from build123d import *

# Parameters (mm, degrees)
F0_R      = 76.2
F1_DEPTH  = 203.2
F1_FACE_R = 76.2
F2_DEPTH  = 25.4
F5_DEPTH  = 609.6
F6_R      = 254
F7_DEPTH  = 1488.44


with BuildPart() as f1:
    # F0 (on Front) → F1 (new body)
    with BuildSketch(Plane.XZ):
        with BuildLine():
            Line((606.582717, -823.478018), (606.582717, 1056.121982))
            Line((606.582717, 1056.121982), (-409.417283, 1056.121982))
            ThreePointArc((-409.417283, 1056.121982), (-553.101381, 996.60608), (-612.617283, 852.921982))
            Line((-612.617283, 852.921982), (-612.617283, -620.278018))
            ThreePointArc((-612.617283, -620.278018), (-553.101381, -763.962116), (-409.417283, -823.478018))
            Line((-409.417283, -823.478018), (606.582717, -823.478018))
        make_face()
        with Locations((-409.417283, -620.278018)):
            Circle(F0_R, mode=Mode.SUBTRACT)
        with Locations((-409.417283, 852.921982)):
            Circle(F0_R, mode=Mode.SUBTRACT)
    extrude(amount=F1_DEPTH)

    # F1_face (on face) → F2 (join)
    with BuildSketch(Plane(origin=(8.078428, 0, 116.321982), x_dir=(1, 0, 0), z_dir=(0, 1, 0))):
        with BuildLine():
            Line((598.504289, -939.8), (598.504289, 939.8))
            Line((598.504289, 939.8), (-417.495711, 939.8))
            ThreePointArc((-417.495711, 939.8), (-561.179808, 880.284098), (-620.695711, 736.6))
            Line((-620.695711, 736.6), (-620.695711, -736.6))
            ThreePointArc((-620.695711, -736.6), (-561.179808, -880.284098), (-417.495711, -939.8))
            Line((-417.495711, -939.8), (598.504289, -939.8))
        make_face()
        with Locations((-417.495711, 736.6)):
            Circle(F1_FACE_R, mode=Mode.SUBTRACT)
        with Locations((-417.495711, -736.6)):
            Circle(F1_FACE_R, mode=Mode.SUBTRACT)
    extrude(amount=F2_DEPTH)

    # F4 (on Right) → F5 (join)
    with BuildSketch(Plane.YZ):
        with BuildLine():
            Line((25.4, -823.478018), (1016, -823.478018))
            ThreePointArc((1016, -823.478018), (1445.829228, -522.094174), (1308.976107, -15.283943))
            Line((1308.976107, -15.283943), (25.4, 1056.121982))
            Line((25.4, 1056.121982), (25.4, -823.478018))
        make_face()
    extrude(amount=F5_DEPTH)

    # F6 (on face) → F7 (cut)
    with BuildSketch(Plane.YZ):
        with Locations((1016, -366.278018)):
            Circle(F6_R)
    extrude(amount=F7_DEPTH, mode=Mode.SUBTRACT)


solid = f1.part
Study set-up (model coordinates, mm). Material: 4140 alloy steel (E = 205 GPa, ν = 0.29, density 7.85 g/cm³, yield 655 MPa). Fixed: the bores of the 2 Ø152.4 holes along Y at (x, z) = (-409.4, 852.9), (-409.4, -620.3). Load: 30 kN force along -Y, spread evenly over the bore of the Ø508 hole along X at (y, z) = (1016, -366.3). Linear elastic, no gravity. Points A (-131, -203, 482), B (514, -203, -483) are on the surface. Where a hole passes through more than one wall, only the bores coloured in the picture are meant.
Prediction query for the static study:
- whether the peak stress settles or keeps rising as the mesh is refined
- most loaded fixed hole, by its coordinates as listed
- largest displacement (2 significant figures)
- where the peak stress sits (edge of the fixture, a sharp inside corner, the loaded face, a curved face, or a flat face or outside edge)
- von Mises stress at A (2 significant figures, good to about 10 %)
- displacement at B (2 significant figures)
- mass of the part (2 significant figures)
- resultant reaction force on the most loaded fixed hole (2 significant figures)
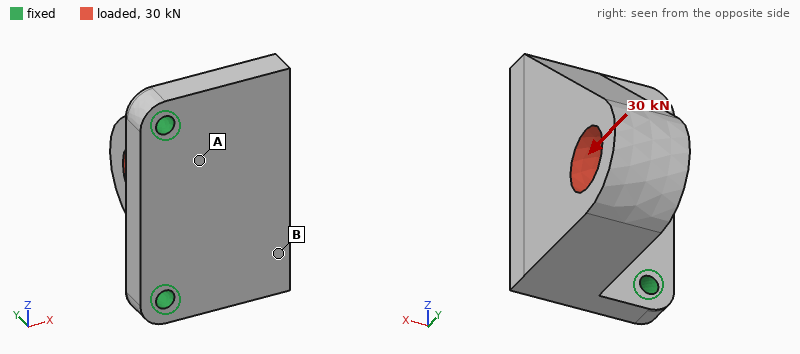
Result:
keeps rising
(-409.4, -620.3)
46 µm
edge of the fixture
0.60 MPa
21 µm
12000 kg
25 kN
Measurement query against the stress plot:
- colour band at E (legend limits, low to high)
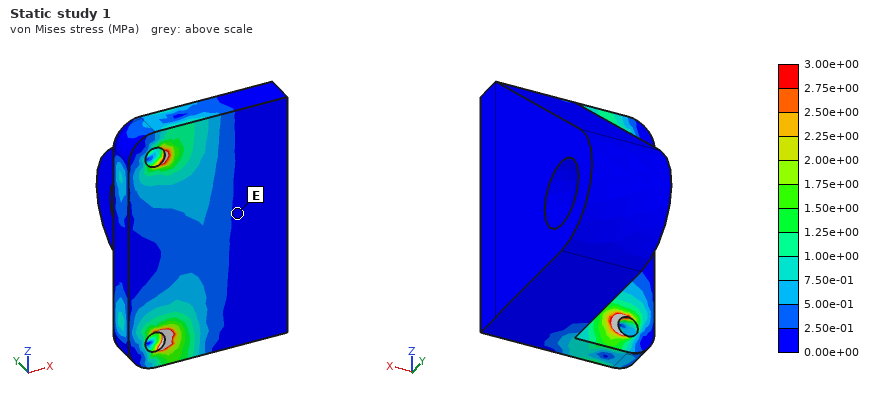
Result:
0.00e+00 to 2.50e-01 MPa
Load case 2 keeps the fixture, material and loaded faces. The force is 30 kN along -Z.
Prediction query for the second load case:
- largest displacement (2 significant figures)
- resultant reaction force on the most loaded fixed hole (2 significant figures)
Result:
11 µm
30 kN
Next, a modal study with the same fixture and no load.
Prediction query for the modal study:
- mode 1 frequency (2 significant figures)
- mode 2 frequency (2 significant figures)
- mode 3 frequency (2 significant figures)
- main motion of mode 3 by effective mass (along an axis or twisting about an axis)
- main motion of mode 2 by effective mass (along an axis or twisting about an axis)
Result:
46 Hz
140 Hz
210 Hz
along Y
along Z
